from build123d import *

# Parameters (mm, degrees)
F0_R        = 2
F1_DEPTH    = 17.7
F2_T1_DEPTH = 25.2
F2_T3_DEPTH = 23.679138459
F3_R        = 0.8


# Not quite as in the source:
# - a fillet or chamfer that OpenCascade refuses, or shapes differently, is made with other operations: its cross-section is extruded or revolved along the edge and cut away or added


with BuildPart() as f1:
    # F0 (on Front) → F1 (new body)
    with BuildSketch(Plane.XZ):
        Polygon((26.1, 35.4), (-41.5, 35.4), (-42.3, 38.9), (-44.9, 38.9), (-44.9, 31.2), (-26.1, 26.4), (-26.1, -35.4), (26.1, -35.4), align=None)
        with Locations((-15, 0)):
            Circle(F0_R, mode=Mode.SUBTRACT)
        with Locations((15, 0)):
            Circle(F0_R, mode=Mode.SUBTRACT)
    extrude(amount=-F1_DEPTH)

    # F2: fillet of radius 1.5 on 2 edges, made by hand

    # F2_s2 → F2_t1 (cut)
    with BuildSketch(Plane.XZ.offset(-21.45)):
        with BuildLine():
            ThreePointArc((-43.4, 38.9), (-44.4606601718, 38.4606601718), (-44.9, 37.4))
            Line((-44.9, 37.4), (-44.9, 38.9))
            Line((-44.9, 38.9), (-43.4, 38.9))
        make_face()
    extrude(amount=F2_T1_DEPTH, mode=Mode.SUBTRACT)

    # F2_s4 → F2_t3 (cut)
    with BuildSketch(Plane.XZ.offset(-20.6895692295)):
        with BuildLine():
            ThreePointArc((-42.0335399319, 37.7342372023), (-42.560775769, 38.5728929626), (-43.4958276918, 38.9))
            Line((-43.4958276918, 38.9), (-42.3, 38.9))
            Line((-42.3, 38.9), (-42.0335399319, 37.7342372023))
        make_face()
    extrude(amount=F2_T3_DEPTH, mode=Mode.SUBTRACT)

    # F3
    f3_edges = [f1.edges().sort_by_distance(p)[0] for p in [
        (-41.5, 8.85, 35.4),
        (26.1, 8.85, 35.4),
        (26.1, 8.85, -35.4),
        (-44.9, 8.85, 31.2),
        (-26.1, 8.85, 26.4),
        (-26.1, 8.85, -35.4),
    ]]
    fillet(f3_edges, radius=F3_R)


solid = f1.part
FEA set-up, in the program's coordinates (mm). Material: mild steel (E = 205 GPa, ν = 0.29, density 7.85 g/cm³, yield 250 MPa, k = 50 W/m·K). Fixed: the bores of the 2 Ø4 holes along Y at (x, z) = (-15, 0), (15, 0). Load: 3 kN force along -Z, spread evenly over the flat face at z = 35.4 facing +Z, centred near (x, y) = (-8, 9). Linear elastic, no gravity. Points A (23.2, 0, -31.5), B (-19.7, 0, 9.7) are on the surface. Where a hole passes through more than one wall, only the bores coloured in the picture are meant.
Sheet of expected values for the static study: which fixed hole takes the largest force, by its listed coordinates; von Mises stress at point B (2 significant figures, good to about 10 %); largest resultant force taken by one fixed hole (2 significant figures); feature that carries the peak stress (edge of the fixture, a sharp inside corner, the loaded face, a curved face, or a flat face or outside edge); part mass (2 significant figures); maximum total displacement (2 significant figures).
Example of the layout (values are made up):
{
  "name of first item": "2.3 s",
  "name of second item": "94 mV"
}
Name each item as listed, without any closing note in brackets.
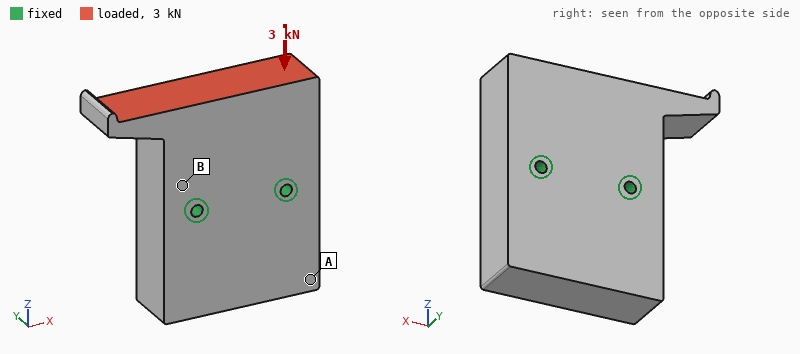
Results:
{
  "which fixed hole takes the largest force, by its listed coordinates": "(-15, 0)",
  "von Mises stress at point B": "6.9 MPa",
  "largest resultant force taken by one fixed hole": "2.2 kN",
  "feature that carries the peak stress": "a curved face",
  "part mass": "530 g",
  "maximum total displacement": "8.3 µm"
}
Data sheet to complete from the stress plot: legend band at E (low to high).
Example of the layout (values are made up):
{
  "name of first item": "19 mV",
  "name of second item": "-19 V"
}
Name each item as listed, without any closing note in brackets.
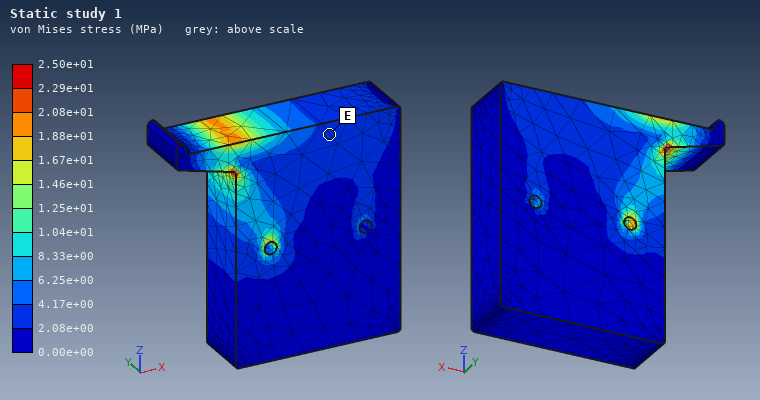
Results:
{
  "legend band at E": "2.08e+00 to 4.17e+00 MPa"
}
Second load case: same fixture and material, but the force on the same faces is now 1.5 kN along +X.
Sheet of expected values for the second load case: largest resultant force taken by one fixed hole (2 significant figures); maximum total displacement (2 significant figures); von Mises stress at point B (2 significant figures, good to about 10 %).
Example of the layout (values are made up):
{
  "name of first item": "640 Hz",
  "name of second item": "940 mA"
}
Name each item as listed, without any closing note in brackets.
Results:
{
  "largest resultant force taken by one fixed hole": "1.8 kN",
  "maximum total displacement": "5.1 µm",
  "von Mises stress at point B": "3.6 MPa"
}
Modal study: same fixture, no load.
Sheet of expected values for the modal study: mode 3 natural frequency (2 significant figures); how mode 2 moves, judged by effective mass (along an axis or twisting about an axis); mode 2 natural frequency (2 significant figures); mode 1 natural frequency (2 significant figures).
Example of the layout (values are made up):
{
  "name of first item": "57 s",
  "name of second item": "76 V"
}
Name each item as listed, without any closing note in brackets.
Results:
{
  "mode 3 natural frequency": "11 kHz",
  "how mode 2 moves, judged by effective mass": "along Y",
  "mode 2 natural frequency": "9200 Hz",
  "mode 1 natural frequency": "6800 Hz"
}
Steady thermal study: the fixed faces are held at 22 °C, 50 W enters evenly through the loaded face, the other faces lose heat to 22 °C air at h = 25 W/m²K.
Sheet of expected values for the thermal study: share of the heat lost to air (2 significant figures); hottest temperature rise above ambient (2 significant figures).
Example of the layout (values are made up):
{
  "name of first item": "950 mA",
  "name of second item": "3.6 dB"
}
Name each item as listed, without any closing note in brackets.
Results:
{
  "share of the heat lost to air": "8.0 %",
  "hottest temperature rise above ambient": "58 K"
}
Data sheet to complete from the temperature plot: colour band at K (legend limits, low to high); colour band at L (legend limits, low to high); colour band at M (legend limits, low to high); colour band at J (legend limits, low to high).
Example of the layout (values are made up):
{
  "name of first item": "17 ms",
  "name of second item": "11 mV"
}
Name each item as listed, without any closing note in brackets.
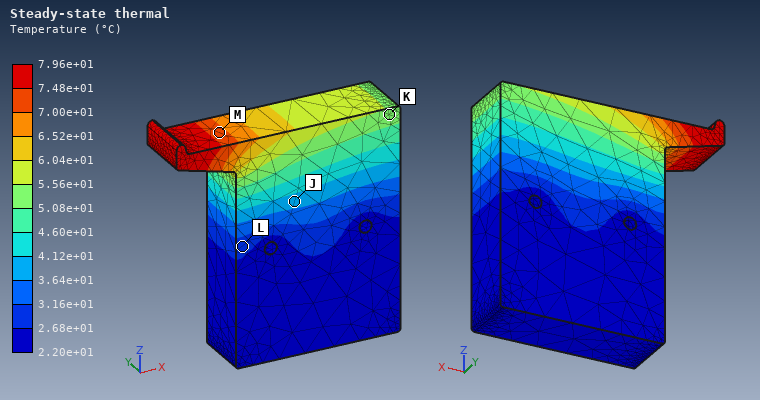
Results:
{
  "colour band at K": "5.08e+01 to 5.56e+01 °C",
  "colour band at L": "2.68e+01 to 3.16e+01 °C",
  "colour band at M": "7.00e+01 to 7.48e+01 °C",
  "colour band at J": "3.64e+01 to 4.12e+01 °C"
}
